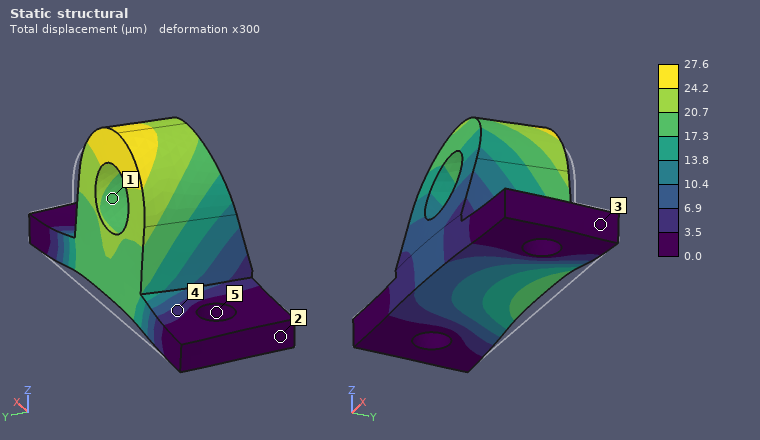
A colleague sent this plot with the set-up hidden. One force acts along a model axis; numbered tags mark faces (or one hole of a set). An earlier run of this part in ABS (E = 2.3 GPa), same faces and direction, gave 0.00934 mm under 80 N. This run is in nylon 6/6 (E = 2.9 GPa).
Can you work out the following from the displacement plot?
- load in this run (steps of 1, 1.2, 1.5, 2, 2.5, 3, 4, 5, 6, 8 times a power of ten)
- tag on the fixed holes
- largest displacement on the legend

300 N
5
27.6 µm
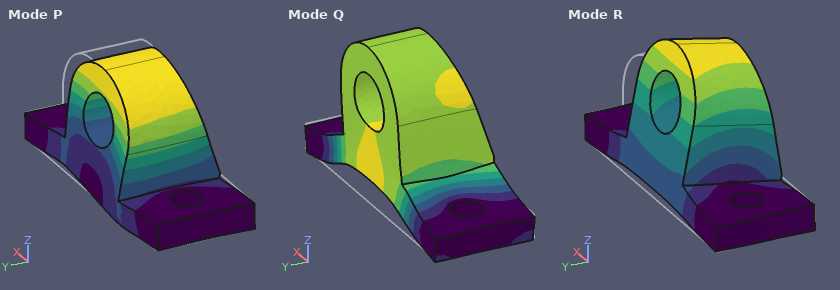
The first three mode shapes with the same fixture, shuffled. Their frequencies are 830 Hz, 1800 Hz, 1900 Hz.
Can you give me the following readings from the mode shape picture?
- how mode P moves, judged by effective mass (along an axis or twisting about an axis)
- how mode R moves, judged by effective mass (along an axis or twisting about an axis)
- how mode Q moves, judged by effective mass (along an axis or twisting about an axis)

along X
along Y
along Z
